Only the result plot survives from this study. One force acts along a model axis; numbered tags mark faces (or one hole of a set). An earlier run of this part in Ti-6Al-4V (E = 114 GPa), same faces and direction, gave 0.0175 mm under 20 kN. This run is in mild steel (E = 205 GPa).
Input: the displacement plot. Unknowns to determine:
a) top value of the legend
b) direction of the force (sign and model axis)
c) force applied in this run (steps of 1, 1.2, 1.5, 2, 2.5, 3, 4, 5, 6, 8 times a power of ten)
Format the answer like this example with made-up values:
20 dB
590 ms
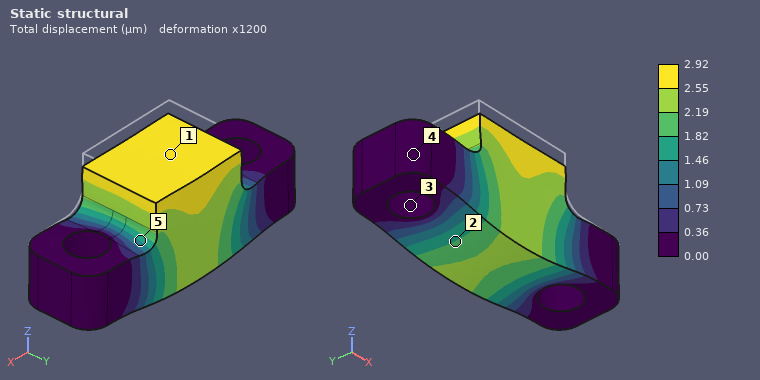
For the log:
2.92 µm
-Z
6 kN
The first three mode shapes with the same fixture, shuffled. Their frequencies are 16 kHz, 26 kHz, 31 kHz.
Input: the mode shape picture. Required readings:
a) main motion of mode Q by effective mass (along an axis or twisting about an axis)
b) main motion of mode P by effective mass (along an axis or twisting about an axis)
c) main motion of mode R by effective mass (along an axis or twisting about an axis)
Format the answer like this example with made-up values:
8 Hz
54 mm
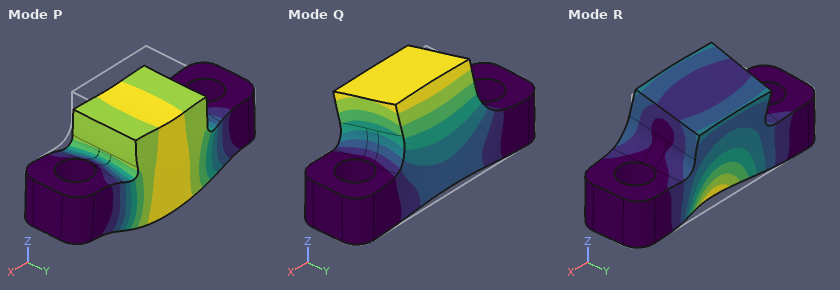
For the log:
along Y
along Z
along Y
